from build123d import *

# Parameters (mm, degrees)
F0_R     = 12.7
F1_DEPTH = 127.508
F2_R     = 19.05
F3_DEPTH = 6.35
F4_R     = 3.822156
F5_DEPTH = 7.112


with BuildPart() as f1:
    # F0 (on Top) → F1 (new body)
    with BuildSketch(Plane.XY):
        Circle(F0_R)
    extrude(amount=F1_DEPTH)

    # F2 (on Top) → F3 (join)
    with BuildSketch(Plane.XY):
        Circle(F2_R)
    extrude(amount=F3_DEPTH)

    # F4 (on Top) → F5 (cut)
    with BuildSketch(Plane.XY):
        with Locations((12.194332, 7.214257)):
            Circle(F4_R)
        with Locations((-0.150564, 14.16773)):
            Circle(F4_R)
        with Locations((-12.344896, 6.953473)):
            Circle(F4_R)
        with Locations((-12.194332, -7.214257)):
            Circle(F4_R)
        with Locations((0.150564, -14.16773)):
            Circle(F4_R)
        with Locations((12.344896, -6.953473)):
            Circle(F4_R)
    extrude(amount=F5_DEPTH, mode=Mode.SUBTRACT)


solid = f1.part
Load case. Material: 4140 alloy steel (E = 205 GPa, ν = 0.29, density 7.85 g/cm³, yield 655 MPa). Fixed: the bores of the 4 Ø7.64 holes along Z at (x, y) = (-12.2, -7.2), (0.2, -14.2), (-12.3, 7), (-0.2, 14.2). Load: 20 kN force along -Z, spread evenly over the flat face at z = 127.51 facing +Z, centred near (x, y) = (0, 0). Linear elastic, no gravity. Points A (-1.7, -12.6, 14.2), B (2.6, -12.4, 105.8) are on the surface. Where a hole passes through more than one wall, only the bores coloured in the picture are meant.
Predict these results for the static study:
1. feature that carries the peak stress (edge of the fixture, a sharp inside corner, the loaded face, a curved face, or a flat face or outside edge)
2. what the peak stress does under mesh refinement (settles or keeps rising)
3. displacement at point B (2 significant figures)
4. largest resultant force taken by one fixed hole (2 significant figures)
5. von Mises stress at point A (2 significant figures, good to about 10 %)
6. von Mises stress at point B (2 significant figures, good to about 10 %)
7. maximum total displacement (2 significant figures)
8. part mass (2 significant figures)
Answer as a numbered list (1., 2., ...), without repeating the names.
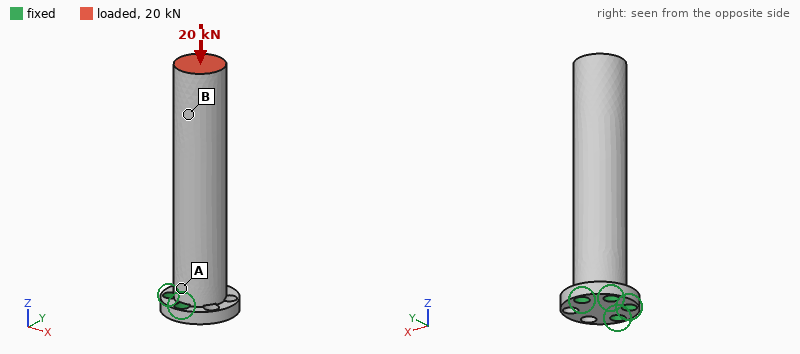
1. edge of the fixture
2. keeps rising
3. 43 µm
4. 8.0 kN
5. 60 MPa
6. 39 MPa
7. 55 µm
8. 520 g
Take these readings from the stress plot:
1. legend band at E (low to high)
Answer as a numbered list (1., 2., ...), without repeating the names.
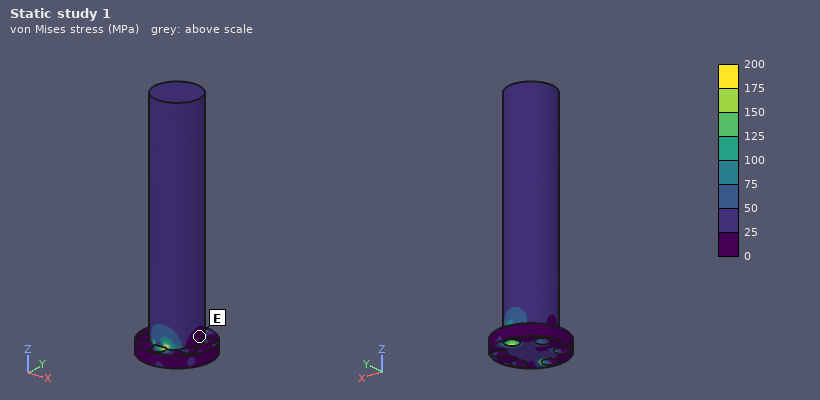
1. 0 to 25 MPa
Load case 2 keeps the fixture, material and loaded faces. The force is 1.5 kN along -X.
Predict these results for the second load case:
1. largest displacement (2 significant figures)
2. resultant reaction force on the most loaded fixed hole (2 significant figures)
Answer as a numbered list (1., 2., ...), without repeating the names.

1. 0.30 mm
2. 6.3 kN
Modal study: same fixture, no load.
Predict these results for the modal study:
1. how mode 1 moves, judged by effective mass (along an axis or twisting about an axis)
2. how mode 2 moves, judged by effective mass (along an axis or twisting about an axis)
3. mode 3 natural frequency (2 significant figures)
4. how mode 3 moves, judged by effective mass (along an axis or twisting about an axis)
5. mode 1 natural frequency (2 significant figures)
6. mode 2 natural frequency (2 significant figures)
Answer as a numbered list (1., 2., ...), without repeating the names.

1. along X
2. along Y
3. 5900 Hz
4. along X
5. 1000 Hz
6. 1100 Hz
